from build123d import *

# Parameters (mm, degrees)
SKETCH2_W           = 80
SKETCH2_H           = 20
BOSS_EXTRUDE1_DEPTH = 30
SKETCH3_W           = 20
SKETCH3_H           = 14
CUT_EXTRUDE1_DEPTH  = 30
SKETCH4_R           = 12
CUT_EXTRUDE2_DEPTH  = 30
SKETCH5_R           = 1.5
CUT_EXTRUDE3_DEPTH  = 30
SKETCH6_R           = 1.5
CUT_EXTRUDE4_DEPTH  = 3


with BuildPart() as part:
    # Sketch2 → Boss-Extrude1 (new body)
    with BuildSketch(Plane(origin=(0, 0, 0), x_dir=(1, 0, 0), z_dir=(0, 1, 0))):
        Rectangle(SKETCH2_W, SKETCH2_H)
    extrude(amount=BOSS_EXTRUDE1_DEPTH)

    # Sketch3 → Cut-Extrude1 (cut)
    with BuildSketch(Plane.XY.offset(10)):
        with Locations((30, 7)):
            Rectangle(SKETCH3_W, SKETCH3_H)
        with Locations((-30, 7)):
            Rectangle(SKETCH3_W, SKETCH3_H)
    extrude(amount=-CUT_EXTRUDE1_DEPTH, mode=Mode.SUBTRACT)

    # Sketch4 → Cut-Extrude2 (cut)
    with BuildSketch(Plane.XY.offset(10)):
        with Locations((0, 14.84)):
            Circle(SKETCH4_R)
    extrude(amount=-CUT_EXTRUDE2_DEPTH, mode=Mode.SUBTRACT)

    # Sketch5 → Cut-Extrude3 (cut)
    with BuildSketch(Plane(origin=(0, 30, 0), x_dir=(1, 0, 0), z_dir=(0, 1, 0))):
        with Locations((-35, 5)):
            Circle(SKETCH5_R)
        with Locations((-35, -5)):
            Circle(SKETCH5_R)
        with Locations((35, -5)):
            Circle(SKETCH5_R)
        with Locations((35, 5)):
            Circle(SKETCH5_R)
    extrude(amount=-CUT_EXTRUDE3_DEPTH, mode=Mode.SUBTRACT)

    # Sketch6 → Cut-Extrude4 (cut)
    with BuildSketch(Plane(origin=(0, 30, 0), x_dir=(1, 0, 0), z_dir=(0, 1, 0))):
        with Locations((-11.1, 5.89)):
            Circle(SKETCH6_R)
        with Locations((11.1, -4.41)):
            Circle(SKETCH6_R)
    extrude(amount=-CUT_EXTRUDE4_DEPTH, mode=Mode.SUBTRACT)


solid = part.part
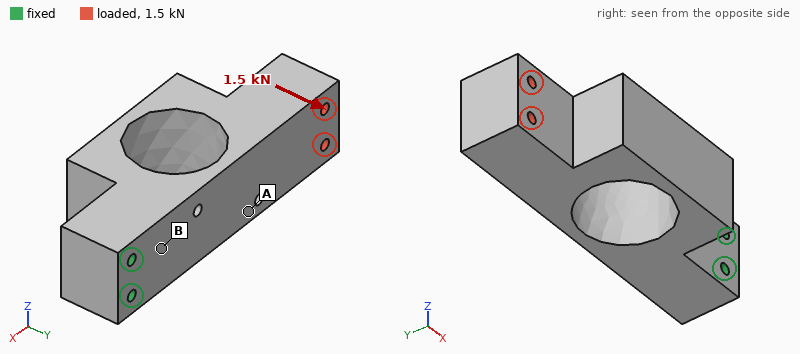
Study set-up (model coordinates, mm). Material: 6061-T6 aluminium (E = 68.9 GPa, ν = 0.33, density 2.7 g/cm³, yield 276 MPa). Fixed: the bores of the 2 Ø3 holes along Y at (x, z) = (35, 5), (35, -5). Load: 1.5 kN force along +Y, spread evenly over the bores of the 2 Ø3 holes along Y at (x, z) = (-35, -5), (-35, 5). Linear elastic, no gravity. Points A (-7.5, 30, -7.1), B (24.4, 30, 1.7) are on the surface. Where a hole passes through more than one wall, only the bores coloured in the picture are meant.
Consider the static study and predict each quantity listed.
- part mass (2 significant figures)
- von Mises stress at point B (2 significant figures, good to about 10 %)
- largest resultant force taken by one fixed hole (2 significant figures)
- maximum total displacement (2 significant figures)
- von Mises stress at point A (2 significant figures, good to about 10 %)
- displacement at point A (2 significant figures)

74 g
100 MPa
750 N
0.49 mm
30 MPa
0.23 mm
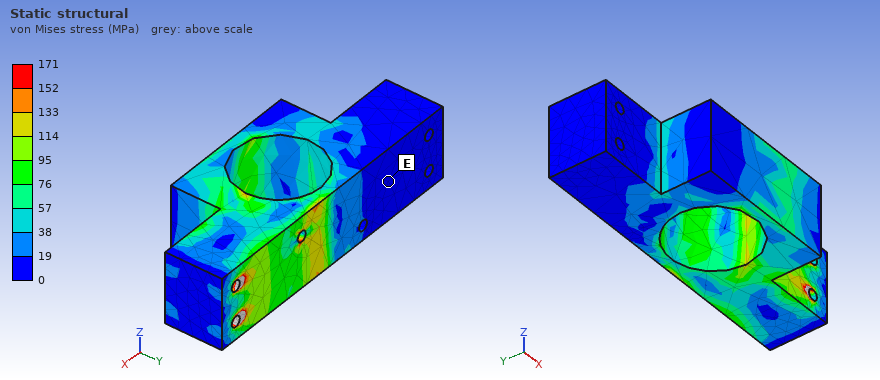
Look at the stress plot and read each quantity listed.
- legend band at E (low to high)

0 to 19 MPa
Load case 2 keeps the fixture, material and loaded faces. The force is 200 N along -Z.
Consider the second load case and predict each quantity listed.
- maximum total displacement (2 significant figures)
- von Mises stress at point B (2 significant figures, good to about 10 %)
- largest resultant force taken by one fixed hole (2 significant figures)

61 µm
2.9 MPa
1.2 kN
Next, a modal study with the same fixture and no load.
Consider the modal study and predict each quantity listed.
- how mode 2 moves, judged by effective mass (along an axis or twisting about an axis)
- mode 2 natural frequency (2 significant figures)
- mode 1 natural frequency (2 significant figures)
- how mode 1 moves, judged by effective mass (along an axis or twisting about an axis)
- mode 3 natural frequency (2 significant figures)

along Z
2200 Hz
1900 Hz
along Y
6000 Hz
